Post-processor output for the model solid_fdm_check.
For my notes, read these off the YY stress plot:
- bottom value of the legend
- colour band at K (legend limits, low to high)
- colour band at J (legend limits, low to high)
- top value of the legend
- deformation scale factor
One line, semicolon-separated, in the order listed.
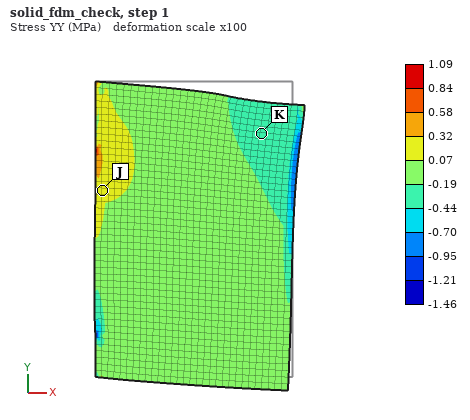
-1.46 MPa; -0.44 to -0.19 MPa; 0.07 to 0.32 MPa; 1.09 MPa; 100
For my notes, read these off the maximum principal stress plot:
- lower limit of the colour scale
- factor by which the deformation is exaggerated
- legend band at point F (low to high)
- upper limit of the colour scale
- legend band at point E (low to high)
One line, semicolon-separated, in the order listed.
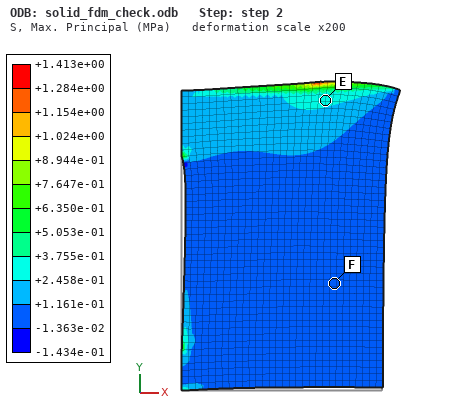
-1.434e-01 MPa; 200; -1.363e-02 to +1.161e-01 MPa; +1.413e+00 MPa; +2.458e-01 to +3.755e-01 MPa
